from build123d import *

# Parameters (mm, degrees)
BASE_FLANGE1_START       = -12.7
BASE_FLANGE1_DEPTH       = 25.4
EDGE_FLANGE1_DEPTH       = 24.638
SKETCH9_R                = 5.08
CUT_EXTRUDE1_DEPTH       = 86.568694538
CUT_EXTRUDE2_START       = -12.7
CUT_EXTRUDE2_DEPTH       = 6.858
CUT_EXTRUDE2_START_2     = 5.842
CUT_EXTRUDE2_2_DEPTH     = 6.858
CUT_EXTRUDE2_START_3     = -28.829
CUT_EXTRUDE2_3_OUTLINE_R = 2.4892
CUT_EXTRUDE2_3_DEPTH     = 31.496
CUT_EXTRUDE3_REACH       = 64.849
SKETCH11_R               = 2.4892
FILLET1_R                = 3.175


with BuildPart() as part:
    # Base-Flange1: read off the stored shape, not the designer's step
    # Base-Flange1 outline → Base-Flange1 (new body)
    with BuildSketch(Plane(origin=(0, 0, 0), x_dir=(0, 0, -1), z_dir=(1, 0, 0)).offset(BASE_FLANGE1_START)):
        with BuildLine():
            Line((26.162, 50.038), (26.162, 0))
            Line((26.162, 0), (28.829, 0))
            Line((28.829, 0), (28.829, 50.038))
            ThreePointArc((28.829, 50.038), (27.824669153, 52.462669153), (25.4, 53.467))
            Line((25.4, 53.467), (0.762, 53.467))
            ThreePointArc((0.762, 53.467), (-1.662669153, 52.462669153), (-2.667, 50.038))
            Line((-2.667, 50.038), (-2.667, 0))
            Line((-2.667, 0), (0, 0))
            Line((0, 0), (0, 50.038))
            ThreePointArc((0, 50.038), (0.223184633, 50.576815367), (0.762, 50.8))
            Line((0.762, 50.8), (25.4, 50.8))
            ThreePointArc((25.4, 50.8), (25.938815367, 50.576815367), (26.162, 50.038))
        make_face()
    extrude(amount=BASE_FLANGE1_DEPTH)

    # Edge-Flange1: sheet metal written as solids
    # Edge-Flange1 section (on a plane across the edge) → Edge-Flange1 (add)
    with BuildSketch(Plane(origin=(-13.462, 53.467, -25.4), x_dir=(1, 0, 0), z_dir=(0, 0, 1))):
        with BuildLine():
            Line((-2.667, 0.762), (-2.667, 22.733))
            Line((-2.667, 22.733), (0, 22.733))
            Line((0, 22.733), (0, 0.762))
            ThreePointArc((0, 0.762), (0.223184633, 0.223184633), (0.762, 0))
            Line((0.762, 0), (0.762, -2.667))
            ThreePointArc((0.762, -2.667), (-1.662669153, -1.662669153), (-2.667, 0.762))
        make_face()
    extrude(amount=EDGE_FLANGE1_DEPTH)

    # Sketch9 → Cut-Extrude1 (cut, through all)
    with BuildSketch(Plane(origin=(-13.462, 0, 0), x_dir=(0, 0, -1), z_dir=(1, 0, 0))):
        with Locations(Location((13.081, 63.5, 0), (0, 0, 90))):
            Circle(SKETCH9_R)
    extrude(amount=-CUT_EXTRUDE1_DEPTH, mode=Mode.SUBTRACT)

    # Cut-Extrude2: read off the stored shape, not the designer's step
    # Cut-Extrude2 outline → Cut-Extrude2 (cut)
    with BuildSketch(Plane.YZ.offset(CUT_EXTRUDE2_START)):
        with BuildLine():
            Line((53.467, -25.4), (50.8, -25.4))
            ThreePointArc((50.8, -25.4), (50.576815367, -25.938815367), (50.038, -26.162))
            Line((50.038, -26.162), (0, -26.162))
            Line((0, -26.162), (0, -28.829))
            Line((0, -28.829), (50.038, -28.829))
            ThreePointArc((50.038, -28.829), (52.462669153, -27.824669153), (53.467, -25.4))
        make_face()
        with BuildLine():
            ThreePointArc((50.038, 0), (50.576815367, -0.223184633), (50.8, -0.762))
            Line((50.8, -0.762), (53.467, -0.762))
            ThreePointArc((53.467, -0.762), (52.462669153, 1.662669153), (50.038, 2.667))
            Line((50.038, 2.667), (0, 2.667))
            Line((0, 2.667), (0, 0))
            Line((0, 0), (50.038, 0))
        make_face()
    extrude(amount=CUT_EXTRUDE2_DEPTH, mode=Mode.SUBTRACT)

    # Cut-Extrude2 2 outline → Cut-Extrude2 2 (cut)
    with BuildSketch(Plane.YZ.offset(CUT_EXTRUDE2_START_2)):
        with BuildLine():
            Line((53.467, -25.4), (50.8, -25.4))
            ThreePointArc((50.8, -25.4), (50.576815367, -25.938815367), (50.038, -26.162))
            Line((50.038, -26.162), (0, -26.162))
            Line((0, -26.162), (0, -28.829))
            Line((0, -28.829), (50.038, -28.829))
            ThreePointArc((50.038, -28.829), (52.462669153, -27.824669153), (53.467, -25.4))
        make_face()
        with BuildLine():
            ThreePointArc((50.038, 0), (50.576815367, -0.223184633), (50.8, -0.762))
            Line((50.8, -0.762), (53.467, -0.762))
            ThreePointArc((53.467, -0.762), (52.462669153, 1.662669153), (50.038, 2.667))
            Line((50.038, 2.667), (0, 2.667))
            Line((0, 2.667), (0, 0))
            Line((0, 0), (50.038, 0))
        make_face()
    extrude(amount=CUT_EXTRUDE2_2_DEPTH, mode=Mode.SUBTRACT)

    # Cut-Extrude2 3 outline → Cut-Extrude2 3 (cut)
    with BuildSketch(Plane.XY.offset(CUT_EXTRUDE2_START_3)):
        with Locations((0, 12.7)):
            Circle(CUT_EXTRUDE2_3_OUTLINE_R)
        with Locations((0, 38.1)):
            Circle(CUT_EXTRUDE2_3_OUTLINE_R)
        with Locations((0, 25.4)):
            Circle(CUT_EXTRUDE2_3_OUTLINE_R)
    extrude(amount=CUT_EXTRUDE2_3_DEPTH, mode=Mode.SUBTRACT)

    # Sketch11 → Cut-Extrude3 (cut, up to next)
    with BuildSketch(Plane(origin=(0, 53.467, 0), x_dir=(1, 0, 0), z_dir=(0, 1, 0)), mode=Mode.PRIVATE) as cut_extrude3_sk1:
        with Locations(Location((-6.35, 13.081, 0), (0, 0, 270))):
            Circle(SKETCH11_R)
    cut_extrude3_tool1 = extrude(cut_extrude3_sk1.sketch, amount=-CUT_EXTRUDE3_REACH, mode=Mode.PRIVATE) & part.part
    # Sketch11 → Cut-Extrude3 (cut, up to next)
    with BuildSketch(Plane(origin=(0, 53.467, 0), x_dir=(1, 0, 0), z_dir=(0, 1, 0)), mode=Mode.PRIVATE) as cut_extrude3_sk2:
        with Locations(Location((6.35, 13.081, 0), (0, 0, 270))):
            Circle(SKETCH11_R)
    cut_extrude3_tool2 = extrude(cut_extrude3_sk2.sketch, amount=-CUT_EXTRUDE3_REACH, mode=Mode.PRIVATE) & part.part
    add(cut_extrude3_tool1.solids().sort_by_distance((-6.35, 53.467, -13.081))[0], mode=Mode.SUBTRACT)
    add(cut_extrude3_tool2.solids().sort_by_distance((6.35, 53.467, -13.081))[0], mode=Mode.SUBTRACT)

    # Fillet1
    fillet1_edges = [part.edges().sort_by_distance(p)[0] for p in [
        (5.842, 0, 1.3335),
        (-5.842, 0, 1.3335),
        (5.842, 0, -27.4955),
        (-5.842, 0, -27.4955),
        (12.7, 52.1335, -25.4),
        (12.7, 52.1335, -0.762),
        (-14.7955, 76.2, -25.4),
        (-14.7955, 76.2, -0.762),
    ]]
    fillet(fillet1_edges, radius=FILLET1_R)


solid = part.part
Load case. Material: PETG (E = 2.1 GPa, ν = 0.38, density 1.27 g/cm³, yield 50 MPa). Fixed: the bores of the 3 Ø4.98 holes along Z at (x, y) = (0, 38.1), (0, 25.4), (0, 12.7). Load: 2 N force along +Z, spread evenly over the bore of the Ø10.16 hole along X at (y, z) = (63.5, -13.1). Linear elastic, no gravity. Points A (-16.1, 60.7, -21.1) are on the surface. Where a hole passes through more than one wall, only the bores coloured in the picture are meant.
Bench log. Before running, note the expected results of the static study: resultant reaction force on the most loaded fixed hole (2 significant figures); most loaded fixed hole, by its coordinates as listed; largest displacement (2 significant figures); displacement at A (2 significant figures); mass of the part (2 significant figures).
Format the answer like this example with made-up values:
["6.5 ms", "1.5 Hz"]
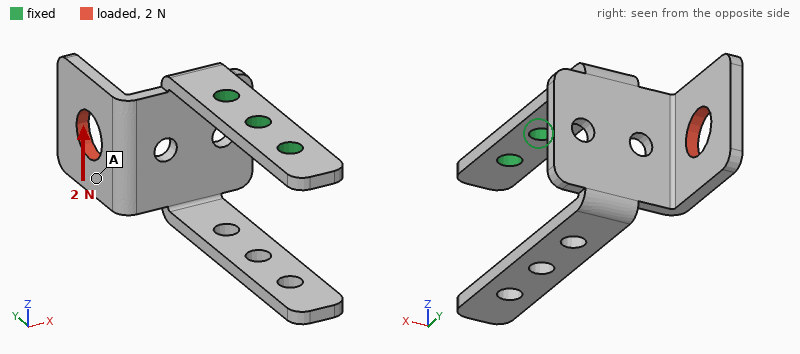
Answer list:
["2.0 N", "(0, 38.1)", "0.92 mm", "0.49 mm", "7.6 g"]
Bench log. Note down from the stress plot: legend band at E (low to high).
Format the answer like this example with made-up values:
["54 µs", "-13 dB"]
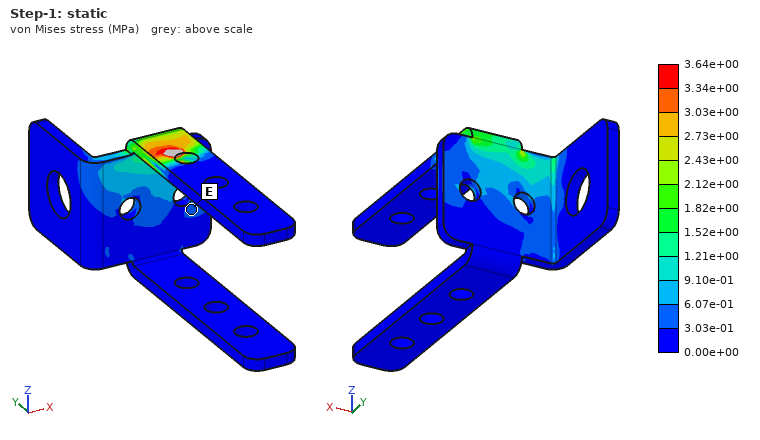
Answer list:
["3.03e-01 to 6.07e-01 MPa"]
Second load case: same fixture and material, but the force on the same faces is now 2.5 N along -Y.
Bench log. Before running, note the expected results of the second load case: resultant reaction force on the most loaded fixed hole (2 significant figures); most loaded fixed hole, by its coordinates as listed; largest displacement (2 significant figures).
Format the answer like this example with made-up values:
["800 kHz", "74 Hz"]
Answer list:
["2.5 N", "(0, 38.1)", "0.94 mm"]
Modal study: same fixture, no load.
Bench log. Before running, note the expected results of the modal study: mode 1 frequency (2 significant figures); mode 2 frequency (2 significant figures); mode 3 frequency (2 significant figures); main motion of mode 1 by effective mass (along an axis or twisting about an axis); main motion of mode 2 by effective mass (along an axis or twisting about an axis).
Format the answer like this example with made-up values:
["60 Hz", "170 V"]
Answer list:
["100 Hz", "150 Hz", "220 Hz", "along Y", "along X"]
